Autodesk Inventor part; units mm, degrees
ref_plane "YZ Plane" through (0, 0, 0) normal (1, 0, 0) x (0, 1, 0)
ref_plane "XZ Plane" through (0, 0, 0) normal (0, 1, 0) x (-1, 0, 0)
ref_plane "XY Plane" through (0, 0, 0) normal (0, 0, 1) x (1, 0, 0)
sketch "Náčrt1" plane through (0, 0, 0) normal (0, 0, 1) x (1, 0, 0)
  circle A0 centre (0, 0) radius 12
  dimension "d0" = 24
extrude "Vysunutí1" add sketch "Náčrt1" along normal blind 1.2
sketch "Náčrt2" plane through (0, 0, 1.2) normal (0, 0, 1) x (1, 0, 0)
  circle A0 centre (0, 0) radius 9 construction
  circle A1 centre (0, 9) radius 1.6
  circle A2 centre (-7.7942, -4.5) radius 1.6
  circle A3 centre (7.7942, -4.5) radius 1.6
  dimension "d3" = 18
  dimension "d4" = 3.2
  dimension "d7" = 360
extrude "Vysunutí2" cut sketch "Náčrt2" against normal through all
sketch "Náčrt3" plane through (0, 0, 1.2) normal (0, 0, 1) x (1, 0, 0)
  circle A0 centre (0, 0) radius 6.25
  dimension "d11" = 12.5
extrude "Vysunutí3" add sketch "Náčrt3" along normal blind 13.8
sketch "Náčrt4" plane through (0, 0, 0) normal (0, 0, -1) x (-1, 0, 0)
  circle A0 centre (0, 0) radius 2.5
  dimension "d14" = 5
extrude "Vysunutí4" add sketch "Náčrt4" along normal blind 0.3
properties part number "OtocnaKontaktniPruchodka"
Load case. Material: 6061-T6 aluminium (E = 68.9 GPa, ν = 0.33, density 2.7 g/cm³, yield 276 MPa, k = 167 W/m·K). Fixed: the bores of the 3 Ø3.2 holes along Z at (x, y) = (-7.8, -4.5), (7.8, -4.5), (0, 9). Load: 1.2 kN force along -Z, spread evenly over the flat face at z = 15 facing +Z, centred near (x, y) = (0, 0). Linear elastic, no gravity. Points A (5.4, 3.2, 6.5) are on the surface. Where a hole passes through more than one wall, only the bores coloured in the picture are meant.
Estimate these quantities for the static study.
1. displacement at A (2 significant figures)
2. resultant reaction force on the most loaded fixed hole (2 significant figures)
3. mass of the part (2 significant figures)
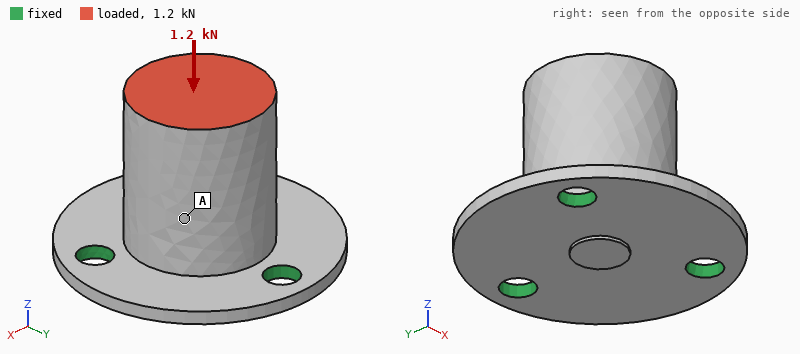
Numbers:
12 µm
440 N
6.0 g
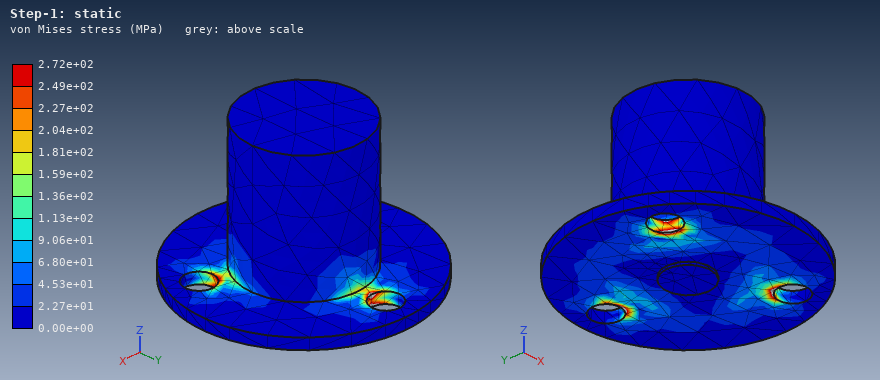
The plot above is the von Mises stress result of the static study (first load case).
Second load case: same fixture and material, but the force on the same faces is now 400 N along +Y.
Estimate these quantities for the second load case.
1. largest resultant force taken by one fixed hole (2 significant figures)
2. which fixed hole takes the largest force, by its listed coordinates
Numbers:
570 N
(0, 9)
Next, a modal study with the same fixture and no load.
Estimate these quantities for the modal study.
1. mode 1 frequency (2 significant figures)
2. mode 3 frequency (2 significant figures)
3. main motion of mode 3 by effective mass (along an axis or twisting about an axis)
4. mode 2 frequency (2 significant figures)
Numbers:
12 kHz
21 kHz
along Z
12 kHz
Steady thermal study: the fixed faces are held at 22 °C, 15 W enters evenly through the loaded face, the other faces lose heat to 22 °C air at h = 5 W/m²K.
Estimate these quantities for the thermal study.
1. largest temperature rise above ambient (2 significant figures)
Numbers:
19 K
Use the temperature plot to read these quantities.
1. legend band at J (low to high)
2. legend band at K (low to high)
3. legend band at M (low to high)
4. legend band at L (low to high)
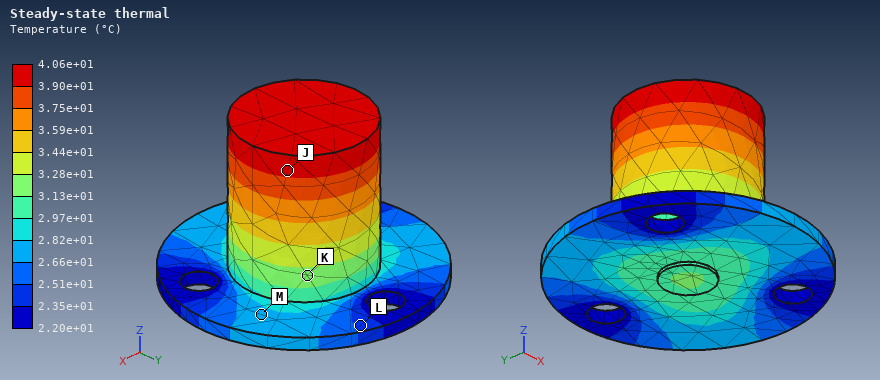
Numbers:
3.90e+01 to 4.06e+01 °C
3.13e+01 to 3.28e+01 °C
2.66e+01 to 2.82e+01 °C
2.35e+01 to 2.51e+01 °C
